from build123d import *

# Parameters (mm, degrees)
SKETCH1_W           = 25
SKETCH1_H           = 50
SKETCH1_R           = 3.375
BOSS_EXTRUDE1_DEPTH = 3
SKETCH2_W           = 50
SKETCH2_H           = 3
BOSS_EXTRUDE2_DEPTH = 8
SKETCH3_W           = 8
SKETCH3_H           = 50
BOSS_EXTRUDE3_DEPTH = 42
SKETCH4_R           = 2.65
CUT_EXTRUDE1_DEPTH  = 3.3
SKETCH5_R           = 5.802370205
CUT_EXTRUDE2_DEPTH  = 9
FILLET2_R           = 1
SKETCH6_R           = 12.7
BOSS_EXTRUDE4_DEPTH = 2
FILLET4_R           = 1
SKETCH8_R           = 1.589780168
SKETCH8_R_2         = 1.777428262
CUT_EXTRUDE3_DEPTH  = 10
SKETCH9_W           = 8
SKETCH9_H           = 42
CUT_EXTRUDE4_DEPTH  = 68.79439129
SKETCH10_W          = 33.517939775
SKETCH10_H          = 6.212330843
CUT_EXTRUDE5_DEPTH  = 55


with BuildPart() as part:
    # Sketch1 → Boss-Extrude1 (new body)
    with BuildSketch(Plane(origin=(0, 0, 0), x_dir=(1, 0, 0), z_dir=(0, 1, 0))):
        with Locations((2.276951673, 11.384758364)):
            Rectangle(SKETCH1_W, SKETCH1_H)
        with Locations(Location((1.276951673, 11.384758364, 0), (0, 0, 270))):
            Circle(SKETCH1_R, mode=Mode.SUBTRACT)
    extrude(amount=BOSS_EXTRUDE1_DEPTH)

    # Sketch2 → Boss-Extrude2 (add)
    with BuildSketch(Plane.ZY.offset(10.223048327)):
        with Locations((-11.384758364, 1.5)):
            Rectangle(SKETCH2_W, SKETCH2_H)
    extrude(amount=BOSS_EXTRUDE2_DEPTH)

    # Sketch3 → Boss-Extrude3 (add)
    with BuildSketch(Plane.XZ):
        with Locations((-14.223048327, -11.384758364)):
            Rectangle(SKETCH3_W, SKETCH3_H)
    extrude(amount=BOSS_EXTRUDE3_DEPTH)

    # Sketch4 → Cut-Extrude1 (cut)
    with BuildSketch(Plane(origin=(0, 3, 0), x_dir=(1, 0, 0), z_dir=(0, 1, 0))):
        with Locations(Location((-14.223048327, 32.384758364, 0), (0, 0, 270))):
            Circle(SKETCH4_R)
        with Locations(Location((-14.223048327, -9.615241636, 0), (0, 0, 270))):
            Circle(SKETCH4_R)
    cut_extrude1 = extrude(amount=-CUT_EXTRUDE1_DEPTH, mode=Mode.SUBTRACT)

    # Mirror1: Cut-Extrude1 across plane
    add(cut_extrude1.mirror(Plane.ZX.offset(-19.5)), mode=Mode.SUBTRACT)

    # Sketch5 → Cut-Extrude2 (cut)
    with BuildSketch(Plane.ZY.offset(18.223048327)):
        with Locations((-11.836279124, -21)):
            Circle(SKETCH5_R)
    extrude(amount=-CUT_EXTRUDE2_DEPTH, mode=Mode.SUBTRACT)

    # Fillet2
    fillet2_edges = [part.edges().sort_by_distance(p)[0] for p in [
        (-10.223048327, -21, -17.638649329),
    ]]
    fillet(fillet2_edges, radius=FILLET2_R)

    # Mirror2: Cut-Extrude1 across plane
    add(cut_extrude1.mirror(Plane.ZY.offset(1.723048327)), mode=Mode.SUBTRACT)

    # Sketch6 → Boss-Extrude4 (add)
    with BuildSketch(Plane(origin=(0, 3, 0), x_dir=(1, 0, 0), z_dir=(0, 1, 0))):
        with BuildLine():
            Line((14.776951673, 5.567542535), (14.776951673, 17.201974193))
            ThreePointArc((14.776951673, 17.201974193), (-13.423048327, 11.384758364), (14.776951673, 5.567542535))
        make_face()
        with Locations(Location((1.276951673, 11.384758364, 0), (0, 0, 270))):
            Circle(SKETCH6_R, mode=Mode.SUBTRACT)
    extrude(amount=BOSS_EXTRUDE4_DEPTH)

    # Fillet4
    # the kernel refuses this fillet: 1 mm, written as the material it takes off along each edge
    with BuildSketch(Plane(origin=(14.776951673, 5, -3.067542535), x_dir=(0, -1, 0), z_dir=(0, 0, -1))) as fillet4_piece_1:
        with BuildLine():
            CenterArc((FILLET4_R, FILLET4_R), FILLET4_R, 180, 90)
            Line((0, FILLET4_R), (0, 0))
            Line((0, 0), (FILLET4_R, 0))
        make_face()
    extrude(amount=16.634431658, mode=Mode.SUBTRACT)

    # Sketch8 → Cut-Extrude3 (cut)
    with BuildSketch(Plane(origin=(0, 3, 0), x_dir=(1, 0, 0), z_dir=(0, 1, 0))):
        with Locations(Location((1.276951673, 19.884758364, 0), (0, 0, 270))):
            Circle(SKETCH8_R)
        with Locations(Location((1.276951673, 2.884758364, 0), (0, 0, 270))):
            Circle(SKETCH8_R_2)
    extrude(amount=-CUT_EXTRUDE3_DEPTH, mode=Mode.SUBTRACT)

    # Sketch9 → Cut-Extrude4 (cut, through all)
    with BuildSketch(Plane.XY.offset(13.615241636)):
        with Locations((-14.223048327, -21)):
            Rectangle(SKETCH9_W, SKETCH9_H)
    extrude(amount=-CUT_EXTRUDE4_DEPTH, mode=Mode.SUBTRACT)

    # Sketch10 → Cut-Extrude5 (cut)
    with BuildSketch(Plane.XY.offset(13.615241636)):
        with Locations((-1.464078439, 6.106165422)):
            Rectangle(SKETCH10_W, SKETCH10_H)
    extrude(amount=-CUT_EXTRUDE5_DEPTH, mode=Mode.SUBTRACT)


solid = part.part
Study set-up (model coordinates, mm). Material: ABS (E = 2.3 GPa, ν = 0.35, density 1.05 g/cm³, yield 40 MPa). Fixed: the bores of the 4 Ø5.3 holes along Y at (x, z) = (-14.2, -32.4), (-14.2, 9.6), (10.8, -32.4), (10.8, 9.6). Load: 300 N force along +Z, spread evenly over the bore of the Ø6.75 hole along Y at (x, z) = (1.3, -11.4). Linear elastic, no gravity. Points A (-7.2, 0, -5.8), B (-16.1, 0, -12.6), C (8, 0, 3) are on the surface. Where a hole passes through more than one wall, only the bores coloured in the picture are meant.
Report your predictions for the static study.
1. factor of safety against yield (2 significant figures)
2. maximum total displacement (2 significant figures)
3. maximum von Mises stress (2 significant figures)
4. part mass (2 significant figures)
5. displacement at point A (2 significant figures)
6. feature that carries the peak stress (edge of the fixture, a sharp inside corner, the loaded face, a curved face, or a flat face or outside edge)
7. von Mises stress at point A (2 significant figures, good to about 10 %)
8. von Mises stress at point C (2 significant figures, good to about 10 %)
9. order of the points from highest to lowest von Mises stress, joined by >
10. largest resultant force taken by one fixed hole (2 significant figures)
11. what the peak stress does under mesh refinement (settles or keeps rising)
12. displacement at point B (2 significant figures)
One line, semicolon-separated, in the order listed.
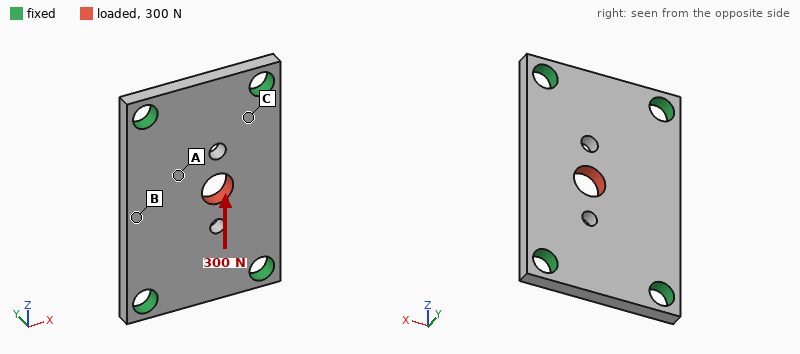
3.9; 31 µm; 10 MPa; 4.8 g; 13 µm; a curved face; 1.7 MPa; 3.2 MPa; C > A > B; 90 N; settles; 5.2 µm
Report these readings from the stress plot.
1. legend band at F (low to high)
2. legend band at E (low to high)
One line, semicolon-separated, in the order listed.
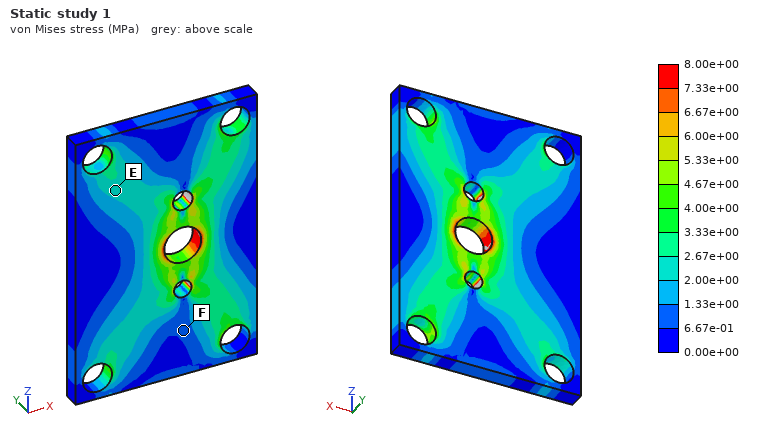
6.67e-01 to 1.33e+00 MPa; 2.00e+00 to 2.67e+00 MPa
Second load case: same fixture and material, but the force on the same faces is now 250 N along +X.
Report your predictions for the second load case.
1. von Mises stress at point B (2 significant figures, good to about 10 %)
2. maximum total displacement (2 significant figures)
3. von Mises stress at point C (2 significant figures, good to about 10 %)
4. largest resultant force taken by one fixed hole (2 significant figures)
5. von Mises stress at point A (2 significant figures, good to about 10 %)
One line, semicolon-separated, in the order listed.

1.6 MPa; 46 µm; 2.5 MPa; 83 N; 2.8 MPa
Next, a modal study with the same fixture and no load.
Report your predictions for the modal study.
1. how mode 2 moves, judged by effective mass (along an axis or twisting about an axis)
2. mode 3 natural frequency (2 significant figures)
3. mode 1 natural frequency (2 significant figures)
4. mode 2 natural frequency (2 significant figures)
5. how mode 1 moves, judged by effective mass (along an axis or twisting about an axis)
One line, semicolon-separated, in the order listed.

twisting about Z; 5900 Hz; 2700 Hz; 3700 Hz; along Y
